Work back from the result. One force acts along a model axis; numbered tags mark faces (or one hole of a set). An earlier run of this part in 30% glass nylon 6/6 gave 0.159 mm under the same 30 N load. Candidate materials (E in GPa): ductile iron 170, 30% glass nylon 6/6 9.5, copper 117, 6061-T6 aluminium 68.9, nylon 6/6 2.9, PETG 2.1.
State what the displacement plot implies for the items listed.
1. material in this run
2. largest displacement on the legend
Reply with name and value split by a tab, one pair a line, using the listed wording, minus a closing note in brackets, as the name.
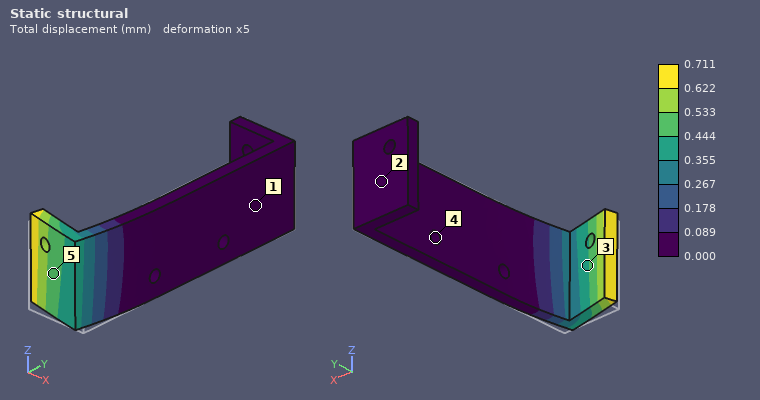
material in this run	PETG
largest displacement on the legend	0.711 mm
